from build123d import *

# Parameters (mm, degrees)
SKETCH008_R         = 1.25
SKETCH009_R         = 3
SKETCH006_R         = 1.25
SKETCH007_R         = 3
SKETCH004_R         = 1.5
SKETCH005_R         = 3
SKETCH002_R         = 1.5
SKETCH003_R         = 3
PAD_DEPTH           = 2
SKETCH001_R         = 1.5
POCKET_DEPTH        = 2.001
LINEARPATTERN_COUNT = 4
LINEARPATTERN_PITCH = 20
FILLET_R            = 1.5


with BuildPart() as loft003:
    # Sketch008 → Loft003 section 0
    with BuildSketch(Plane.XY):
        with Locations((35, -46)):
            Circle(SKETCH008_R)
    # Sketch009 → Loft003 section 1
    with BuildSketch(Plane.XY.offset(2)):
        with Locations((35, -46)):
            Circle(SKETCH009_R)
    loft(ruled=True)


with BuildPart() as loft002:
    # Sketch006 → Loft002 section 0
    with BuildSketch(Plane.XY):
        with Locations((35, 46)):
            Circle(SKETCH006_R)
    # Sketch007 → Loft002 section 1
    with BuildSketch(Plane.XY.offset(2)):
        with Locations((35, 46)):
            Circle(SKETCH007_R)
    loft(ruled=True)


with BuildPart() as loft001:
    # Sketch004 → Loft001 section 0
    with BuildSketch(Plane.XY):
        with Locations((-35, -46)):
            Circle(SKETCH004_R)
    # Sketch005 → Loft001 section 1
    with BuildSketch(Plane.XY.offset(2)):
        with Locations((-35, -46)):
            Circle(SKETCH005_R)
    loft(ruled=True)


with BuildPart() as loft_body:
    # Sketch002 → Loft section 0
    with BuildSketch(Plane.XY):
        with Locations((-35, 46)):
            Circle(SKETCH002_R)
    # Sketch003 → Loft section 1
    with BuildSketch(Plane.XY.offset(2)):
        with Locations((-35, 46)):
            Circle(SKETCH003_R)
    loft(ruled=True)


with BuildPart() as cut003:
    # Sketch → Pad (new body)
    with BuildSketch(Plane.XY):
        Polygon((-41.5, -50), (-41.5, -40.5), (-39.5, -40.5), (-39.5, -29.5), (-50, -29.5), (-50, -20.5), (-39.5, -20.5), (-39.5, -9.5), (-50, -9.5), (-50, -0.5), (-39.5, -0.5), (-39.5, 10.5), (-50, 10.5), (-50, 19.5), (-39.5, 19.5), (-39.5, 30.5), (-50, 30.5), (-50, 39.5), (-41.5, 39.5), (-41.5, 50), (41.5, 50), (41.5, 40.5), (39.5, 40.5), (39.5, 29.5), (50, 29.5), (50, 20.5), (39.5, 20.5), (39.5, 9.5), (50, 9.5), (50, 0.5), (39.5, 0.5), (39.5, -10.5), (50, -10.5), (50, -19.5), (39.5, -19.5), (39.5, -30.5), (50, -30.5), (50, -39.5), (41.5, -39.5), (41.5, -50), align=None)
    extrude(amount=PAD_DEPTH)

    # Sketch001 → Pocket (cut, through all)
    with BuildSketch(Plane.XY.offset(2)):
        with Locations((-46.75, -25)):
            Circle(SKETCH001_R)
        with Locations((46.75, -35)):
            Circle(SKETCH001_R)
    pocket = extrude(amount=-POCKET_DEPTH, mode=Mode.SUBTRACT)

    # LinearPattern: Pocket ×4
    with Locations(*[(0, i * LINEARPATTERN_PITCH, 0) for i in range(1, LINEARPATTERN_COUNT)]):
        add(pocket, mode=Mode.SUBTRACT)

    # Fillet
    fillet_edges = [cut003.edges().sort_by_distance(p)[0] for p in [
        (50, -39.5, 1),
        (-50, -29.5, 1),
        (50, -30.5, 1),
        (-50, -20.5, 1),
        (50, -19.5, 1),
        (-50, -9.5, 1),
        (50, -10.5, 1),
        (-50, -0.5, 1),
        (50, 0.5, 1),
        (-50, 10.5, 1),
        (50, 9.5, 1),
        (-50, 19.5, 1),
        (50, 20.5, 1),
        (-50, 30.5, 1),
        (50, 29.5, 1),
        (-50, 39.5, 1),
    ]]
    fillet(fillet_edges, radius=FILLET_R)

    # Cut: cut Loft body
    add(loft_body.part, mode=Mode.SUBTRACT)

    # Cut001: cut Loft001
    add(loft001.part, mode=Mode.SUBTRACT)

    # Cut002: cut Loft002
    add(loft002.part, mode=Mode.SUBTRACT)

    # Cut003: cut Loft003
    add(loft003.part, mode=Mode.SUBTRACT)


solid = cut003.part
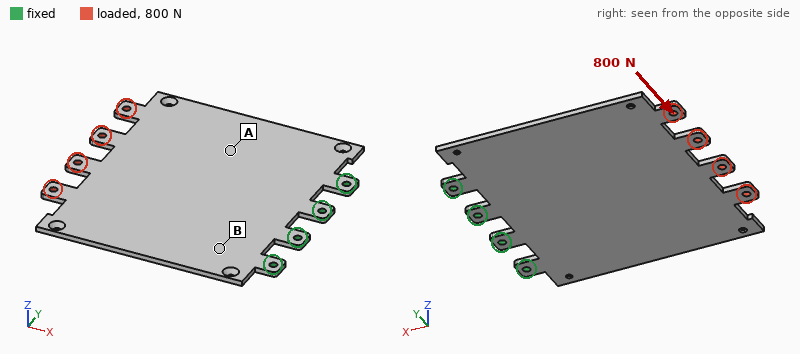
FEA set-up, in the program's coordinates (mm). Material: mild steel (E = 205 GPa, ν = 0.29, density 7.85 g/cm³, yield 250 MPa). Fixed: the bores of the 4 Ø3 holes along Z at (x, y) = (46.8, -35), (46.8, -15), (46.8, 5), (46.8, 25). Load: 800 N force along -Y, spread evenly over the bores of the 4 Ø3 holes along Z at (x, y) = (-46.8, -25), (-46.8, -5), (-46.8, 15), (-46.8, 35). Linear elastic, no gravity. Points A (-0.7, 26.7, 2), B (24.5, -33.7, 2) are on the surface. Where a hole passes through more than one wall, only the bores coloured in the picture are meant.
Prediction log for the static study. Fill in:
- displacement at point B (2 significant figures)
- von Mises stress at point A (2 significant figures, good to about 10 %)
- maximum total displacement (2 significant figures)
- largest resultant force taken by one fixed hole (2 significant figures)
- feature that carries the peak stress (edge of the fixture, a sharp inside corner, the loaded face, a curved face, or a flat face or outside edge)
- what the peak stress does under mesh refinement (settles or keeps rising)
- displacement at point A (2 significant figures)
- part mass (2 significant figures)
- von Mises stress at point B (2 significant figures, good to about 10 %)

7.9 µm
8.7 MPa
35 µm
1.1 kN
edge of the fixture
keeps rising
15 µm
140 g
23 MPa
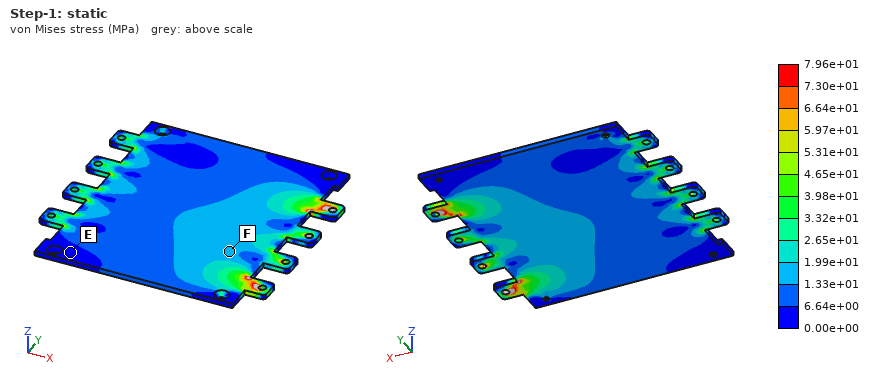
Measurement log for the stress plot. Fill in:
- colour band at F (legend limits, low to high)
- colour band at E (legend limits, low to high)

1.33e+01 to 1.99e+01 MPa
0.00e+00 to 6.64e+00 MPa
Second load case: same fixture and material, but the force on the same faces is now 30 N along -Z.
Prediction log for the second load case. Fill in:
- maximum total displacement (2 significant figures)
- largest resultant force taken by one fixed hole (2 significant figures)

0.92 mm
15 N
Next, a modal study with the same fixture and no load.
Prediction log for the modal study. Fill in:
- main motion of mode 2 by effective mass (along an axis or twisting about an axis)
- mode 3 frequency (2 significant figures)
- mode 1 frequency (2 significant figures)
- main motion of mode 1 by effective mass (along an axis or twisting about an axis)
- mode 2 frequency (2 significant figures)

twisting about X
1000 Hz
160 Hz
along Z
400 Hz
